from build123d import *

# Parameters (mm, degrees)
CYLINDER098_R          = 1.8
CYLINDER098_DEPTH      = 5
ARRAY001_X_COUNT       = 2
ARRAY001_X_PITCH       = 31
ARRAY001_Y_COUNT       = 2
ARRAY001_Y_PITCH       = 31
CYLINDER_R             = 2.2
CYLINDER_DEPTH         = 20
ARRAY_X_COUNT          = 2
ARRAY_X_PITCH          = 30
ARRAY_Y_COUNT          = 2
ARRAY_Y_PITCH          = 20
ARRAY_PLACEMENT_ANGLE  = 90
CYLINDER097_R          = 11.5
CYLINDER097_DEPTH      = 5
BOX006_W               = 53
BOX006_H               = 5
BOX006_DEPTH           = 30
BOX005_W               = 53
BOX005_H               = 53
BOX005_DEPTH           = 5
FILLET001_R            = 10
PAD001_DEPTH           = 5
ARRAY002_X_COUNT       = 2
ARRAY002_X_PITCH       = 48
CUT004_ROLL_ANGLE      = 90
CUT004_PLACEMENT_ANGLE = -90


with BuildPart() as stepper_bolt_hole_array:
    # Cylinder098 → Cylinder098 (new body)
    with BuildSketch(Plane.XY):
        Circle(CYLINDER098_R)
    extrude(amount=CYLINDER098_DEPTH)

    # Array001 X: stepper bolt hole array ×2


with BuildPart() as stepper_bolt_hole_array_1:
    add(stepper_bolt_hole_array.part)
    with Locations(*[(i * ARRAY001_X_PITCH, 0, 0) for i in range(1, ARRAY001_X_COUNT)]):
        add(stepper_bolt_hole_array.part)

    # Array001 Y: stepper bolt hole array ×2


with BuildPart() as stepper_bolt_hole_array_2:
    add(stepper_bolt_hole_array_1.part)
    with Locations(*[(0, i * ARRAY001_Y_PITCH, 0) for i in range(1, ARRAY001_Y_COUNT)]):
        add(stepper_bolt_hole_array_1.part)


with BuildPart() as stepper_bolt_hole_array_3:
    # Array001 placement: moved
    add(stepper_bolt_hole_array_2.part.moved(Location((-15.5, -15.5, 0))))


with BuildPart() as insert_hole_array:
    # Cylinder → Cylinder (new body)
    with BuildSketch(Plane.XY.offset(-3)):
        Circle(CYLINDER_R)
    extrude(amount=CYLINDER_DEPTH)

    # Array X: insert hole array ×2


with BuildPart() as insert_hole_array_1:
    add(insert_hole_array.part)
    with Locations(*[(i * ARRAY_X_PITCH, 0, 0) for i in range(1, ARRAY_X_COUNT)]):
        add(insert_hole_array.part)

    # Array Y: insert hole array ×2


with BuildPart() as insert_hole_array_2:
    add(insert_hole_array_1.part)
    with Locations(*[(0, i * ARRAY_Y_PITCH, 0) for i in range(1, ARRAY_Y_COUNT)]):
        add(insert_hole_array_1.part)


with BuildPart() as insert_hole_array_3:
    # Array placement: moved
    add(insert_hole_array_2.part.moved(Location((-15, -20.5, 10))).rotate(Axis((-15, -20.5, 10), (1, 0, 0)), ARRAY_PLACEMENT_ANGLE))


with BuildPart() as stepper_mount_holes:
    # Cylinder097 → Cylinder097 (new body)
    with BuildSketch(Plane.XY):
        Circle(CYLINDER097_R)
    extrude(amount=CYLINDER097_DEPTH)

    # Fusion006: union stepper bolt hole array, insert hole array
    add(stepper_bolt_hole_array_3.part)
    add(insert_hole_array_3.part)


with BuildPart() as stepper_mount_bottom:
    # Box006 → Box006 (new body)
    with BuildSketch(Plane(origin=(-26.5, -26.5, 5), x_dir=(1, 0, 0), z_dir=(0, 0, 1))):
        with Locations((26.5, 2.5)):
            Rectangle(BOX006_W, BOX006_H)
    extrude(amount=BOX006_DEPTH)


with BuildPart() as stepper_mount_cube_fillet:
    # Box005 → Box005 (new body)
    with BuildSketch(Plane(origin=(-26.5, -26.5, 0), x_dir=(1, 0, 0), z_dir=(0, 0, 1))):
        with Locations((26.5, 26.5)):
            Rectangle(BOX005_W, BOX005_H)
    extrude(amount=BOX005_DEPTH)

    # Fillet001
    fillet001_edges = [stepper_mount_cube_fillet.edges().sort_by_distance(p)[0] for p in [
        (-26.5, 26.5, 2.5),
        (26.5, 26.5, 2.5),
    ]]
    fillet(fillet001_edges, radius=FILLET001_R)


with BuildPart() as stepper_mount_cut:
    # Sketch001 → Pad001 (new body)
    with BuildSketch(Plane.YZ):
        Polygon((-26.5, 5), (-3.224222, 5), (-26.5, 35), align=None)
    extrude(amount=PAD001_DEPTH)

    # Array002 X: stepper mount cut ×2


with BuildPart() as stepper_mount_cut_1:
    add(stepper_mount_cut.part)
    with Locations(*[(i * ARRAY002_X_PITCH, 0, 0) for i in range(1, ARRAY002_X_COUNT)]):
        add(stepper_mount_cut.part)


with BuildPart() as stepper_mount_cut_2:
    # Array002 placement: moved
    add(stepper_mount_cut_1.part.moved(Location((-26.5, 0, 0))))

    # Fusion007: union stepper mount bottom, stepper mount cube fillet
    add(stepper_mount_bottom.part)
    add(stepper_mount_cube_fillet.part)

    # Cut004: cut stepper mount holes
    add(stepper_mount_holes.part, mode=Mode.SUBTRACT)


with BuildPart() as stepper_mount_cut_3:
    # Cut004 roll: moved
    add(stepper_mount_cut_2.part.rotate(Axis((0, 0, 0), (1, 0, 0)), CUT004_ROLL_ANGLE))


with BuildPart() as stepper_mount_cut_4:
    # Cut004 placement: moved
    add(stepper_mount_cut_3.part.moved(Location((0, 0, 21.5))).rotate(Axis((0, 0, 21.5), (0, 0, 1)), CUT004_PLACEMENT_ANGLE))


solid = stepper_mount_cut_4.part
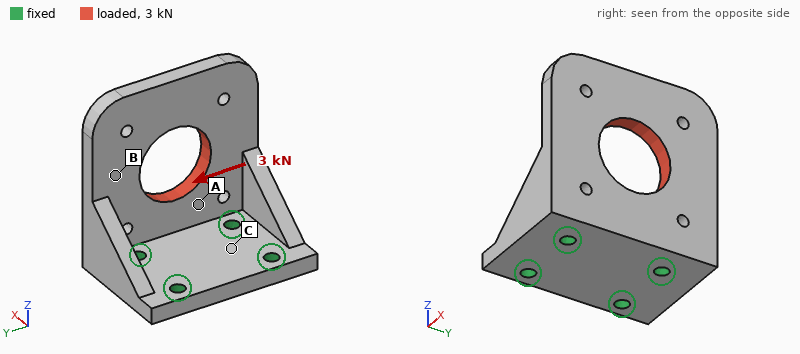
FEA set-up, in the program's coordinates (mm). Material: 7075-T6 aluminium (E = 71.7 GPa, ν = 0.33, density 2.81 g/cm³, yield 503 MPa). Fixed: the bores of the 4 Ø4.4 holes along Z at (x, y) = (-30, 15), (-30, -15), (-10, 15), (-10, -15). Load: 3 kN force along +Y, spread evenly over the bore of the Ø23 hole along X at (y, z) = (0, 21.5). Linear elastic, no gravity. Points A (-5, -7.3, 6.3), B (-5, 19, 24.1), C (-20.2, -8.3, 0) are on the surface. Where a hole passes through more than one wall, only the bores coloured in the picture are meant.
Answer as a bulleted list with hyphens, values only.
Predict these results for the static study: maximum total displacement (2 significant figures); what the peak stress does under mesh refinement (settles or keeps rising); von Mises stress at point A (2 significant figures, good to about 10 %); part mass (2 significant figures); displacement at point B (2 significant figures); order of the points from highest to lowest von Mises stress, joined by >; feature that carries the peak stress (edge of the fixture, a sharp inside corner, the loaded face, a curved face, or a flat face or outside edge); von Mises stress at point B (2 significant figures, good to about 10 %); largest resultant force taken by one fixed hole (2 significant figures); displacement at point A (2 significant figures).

- 0.10 mm
- keeps rising
- 47 MPa
- 60 g
- 0.066 mm
- A > B > C
- edge of the fixture
- 32 MPa
- 2.7 kN
- 0.019 mm
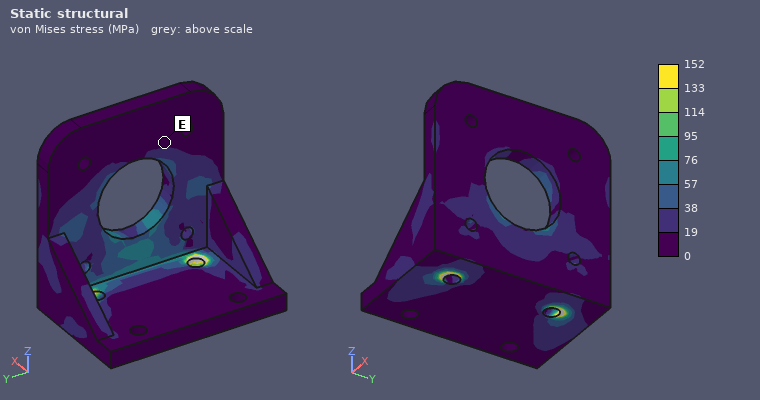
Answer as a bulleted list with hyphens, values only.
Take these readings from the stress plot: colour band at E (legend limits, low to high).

- 0 to 19 MPa
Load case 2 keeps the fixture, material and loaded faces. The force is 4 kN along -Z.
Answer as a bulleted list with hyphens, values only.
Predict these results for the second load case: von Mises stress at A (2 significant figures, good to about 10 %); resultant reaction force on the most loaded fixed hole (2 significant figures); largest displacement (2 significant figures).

- 19 MPa
- 2.4 kN
- 81 µm
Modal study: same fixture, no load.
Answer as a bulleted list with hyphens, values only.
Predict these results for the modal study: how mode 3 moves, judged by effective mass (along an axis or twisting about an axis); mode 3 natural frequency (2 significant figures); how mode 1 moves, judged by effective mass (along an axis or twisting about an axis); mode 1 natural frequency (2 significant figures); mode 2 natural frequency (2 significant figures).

- along Y
- 6300 Hz
- along X
- 2200 Hz
- 4500 Hz
